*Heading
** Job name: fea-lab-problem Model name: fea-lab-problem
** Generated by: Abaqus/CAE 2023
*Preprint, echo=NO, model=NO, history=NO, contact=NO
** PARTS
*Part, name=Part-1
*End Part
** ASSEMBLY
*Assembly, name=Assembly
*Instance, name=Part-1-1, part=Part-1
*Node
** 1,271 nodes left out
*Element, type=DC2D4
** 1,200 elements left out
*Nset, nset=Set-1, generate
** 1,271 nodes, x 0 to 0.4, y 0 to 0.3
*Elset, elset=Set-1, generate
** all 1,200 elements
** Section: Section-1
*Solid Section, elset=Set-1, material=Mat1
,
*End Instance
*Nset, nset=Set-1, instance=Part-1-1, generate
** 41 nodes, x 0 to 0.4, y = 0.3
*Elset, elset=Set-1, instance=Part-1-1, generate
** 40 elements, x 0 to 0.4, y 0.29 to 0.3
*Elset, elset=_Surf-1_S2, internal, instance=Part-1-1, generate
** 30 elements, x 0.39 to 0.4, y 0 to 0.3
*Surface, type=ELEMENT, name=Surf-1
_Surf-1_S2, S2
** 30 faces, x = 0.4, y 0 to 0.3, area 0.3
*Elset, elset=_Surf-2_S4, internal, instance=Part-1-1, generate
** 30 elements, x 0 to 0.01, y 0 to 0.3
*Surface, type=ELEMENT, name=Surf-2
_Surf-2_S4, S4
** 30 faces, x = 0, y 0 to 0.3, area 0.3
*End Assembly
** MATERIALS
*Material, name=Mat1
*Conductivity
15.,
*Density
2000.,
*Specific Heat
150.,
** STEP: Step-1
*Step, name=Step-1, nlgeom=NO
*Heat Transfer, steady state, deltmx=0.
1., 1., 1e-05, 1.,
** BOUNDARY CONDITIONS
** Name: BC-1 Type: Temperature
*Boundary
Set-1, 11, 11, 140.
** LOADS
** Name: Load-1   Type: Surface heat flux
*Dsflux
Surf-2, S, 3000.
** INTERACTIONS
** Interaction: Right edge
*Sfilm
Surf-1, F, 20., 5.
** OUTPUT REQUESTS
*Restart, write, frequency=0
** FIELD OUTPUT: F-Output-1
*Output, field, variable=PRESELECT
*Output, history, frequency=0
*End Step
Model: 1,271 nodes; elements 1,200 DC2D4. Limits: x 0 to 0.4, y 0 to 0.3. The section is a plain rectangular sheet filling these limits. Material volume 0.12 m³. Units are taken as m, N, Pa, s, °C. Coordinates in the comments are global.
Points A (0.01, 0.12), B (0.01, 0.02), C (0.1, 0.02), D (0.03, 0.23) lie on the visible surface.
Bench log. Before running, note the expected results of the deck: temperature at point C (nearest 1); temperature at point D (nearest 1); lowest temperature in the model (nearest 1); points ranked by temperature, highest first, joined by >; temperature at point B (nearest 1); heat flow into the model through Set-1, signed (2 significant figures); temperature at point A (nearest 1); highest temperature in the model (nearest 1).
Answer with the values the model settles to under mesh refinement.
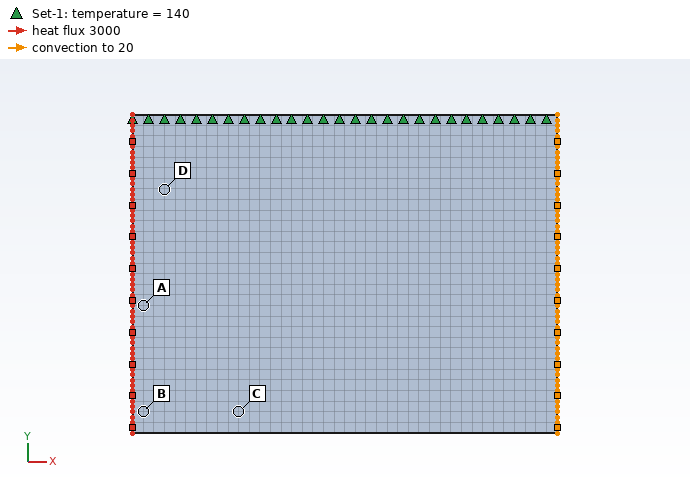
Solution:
167 °C
158 °C
139 °C
B > A > C > D
181 °C
-710 W
177 °C
184 °C
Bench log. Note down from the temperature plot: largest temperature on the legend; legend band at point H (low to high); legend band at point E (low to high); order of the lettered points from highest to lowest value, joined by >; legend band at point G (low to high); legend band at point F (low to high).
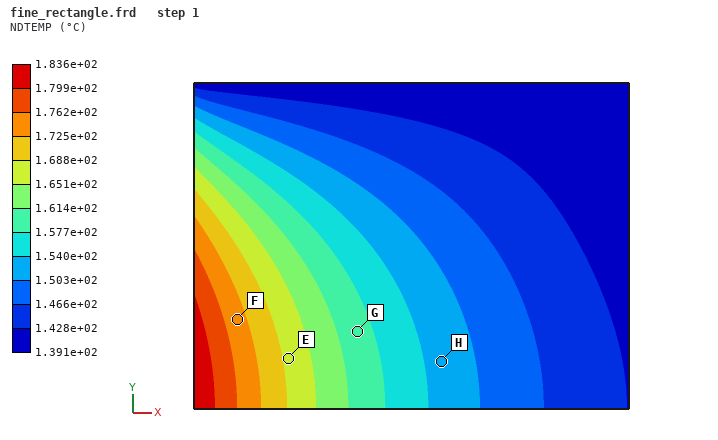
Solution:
1.836e+02 °C
1.503e+02 to 1.540e+02 °C
1.651e+02 to 1.688e+02 °C
F > E > G > H
1.577e+02 to 1.614e+02 °C
1.725e+02 to 1.762e+02 °C
